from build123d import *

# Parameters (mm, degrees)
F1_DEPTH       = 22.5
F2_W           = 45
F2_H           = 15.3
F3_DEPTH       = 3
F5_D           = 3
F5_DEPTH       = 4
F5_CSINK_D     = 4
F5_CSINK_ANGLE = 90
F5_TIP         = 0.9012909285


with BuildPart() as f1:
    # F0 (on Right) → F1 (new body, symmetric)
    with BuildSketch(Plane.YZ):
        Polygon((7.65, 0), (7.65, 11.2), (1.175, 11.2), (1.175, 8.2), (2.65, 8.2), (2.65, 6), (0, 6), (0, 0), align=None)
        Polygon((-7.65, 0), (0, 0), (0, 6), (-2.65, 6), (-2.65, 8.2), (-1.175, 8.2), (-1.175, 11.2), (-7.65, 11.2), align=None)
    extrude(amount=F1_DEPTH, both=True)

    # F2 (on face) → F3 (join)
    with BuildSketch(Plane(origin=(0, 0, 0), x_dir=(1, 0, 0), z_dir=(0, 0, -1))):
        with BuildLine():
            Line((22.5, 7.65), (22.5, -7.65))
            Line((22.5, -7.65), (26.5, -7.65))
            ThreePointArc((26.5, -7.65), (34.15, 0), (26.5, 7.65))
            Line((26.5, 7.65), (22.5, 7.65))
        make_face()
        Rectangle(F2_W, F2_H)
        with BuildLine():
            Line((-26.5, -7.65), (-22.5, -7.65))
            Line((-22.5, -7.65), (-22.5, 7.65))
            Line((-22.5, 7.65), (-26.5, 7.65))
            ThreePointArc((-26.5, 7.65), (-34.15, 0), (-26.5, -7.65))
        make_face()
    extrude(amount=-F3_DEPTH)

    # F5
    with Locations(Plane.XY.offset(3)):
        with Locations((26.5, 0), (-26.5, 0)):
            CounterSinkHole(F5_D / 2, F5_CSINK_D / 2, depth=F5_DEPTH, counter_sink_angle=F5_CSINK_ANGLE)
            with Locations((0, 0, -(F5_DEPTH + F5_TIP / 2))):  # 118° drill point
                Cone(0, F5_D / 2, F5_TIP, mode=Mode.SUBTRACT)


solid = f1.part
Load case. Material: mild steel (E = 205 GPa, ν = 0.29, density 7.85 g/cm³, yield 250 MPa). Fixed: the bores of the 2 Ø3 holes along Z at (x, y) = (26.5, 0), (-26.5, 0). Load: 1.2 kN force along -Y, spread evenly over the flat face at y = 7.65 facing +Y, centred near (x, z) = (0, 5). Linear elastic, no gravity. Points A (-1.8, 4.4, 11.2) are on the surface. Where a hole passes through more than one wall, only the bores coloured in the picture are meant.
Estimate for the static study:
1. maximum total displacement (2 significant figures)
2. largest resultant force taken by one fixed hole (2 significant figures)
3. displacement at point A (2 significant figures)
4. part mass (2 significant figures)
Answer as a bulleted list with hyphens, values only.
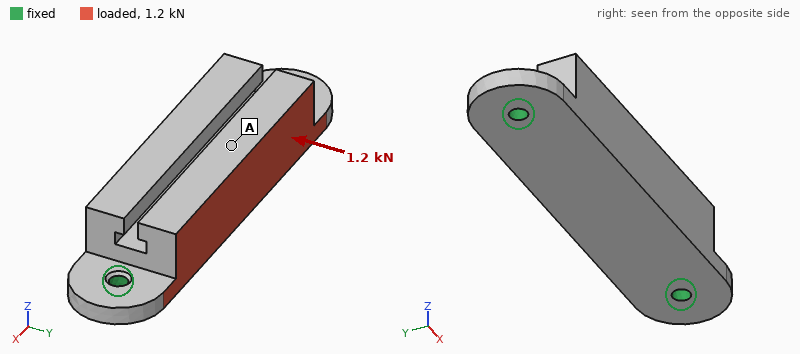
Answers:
- 21 µm
- 600 N
- 19 µm
- 61 g
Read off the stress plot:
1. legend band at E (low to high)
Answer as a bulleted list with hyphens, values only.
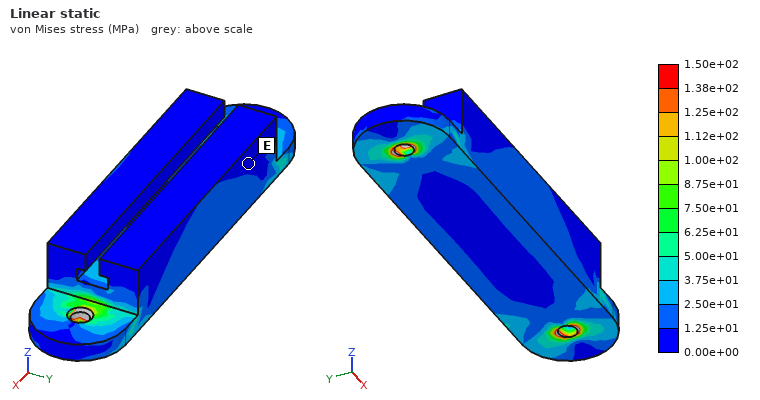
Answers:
- 0.00e+00 to 1.25e+01 MPa
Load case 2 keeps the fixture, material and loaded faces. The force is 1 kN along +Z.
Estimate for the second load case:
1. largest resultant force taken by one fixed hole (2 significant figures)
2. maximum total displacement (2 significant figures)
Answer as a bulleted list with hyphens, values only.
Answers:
- 710 N
- 29 µm
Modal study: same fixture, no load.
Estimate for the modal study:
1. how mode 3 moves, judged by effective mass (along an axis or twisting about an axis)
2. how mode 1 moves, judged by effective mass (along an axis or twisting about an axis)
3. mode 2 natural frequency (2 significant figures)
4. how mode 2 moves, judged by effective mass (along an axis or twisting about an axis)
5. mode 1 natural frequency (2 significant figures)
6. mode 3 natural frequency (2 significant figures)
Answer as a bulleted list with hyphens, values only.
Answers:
- along Y
- along Y
- 9800 Hz
- along Z
- 5900 Hz
- 14 kHz
